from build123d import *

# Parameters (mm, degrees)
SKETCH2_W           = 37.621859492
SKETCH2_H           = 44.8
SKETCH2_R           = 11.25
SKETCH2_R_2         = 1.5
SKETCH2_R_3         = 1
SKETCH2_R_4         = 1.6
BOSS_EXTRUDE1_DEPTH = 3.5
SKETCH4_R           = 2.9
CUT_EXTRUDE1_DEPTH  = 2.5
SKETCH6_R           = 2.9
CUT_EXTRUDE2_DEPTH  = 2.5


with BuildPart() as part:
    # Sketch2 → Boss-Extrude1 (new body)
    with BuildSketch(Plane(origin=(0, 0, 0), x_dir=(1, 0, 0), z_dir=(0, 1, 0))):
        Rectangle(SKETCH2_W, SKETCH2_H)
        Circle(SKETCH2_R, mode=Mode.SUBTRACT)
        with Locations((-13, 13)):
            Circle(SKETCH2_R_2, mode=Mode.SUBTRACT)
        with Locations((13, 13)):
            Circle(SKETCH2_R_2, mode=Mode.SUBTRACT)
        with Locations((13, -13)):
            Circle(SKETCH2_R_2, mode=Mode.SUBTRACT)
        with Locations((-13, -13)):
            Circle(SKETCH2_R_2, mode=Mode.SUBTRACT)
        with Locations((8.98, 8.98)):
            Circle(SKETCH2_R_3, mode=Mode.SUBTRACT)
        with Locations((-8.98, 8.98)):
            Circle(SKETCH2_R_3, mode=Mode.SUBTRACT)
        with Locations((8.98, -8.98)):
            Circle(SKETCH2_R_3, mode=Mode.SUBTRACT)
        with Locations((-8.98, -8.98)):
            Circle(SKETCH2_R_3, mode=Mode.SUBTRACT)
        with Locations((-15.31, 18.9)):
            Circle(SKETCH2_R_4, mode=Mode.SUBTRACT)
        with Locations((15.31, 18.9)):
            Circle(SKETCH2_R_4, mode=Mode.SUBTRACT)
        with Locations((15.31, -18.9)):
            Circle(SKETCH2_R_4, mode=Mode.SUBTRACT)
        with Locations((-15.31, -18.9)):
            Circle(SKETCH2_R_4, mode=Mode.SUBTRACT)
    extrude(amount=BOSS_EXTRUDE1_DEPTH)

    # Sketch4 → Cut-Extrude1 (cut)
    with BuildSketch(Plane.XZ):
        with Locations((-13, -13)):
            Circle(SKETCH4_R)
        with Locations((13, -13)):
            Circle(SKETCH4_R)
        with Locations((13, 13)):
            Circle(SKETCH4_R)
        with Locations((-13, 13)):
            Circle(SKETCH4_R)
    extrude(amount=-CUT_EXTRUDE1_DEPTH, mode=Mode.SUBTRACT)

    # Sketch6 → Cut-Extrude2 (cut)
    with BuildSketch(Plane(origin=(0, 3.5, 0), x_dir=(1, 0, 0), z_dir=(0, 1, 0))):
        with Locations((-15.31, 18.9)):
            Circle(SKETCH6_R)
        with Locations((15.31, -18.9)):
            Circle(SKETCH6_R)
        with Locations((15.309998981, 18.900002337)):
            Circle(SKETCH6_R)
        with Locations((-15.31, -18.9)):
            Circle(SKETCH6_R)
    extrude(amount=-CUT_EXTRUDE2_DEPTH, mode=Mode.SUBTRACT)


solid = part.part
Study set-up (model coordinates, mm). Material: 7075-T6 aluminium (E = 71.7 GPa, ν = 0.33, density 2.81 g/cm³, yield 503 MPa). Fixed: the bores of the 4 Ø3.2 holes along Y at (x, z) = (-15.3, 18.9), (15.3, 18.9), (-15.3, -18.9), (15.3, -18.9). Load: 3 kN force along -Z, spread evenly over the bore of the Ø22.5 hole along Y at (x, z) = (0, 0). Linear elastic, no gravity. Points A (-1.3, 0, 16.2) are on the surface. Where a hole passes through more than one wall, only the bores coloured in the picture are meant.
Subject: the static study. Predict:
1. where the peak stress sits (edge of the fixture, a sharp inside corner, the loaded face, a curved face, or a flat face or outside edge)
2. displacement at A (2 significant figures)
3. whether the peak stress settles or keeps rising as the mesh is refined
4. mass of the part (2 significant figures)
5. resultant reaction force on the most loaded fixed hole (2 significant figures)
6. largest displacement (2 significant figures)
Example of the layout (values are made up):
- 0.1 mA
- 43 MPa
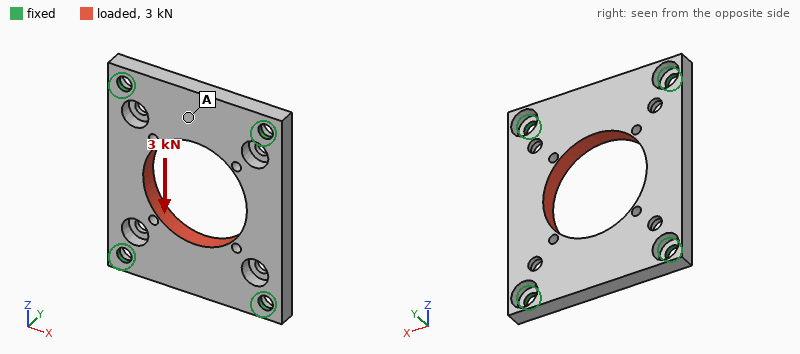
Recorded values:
- edge of the fixture
- 14 µm
- keeps rising
- 11 g
- 760 N
- 18 µm
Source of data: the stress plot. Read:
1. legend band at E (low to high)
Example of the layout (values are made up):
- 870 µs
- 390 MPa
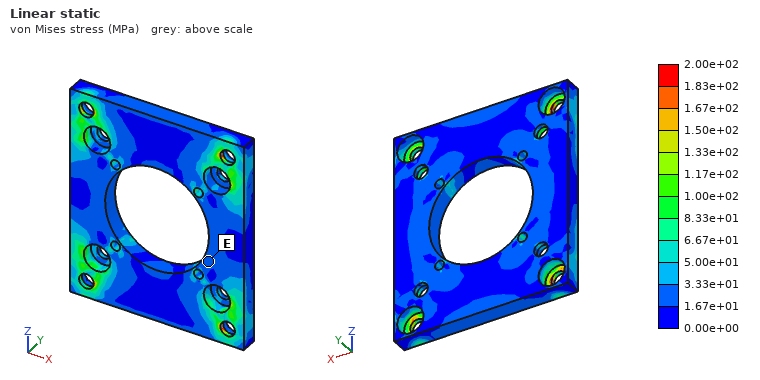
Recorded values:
- 1.67e+01 to 3.33e+01 MPa
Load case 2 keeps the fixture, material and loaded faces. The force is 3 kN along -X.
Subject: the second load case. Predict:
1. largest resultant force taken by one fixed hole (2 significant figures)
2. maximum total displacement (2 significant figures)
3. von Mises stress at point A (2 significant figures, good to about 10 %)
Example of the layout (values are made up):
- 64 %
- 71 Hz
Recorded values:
- 780 N
- 20 µm
- 29 MPa
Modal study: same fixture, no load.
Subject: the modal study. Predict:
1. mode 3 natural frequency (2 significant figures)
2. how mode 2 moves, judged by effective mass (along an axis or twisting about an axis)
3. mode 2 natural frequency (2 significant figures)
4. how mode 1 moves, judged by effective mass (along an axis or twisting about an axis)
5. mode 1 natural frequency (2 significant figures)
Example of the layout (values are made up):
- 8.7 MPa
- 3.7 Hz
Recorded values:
- 13 kHz
- twisting about Z
- 11 kHz
- along Y
- 8200 Hz
